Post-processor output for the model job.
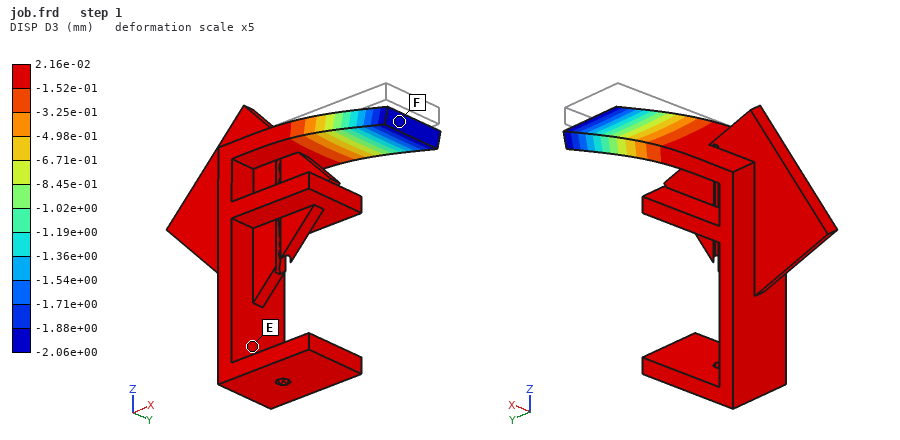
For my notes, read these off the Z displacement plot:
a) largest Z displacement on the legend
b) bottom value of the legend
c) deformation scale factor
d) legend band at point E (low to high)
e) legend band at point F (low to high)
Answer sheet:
2.16e-02 mm
-2.06e+00 mm
5
-1.52e-01 to 2.16e-02 mm
-2.06e+00 to -1.88e+00 mm
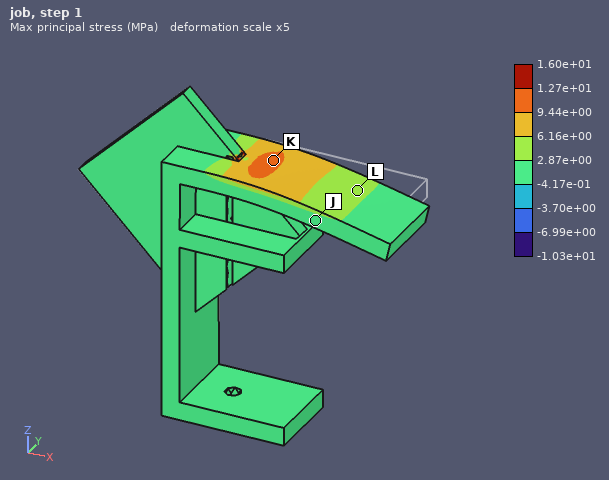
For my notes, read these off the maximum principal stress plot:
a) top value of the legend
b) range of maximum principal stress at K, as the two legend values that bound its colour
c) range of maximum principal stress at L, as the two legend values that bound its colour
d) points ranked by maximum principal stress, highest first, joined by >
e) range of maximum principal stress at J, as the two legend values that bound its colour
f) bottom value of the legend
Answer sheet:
1.60e+01 MPa
9.44e+00 to 1.27e+01 MPa
2.87e+00 to 6.16e+00 MPa
K > L > J
-4.17e-01 to 2.87e+00 MPa
-1.03e+01 MPa
